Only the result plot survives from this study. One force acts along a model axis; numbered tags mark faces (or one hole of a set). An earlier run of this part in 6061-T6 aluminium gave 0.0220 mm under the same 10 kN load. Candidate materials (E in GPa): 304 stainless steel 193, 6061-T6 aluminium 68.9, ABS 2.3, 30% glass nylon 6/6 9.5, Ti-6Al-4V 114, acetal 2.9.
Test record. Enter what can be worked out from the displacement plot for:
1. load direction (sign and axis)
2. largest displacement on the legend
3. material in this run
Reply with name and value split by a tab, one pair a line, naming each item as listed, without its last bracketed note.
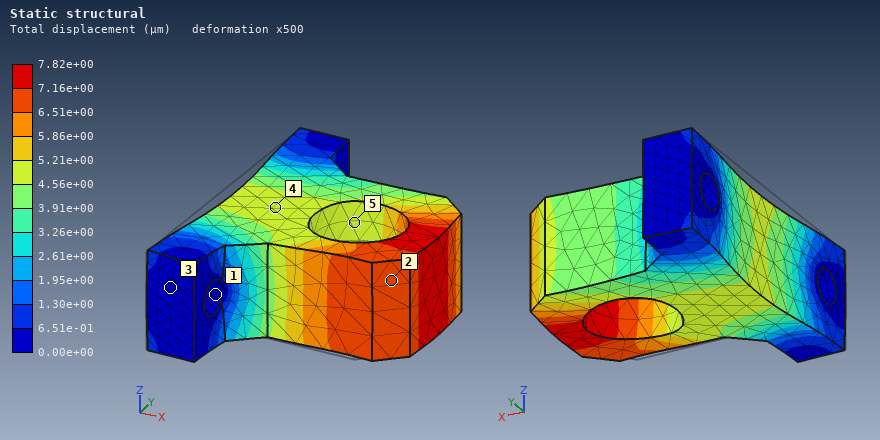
load direction	+X
largest displacement on the legend	7.82e+00 µm
material in this run	304 stainless steel
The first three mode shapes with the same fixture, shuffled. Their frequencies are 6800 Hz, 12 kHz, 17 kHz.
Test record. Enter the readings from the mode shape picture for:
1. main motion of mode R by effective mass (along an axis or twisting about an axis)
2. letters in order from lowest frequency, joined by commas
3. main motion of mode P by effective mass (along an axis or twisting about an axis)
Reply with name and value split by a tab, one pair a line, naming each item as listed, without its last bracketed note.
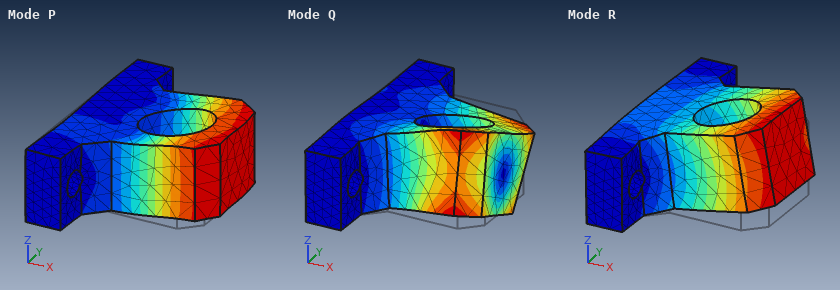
main motion of mode R by effective mass	along Z
letters in order from lowest frequency, joined by commas	R, P, Q
main motion of mode P by effective mass	along Y
